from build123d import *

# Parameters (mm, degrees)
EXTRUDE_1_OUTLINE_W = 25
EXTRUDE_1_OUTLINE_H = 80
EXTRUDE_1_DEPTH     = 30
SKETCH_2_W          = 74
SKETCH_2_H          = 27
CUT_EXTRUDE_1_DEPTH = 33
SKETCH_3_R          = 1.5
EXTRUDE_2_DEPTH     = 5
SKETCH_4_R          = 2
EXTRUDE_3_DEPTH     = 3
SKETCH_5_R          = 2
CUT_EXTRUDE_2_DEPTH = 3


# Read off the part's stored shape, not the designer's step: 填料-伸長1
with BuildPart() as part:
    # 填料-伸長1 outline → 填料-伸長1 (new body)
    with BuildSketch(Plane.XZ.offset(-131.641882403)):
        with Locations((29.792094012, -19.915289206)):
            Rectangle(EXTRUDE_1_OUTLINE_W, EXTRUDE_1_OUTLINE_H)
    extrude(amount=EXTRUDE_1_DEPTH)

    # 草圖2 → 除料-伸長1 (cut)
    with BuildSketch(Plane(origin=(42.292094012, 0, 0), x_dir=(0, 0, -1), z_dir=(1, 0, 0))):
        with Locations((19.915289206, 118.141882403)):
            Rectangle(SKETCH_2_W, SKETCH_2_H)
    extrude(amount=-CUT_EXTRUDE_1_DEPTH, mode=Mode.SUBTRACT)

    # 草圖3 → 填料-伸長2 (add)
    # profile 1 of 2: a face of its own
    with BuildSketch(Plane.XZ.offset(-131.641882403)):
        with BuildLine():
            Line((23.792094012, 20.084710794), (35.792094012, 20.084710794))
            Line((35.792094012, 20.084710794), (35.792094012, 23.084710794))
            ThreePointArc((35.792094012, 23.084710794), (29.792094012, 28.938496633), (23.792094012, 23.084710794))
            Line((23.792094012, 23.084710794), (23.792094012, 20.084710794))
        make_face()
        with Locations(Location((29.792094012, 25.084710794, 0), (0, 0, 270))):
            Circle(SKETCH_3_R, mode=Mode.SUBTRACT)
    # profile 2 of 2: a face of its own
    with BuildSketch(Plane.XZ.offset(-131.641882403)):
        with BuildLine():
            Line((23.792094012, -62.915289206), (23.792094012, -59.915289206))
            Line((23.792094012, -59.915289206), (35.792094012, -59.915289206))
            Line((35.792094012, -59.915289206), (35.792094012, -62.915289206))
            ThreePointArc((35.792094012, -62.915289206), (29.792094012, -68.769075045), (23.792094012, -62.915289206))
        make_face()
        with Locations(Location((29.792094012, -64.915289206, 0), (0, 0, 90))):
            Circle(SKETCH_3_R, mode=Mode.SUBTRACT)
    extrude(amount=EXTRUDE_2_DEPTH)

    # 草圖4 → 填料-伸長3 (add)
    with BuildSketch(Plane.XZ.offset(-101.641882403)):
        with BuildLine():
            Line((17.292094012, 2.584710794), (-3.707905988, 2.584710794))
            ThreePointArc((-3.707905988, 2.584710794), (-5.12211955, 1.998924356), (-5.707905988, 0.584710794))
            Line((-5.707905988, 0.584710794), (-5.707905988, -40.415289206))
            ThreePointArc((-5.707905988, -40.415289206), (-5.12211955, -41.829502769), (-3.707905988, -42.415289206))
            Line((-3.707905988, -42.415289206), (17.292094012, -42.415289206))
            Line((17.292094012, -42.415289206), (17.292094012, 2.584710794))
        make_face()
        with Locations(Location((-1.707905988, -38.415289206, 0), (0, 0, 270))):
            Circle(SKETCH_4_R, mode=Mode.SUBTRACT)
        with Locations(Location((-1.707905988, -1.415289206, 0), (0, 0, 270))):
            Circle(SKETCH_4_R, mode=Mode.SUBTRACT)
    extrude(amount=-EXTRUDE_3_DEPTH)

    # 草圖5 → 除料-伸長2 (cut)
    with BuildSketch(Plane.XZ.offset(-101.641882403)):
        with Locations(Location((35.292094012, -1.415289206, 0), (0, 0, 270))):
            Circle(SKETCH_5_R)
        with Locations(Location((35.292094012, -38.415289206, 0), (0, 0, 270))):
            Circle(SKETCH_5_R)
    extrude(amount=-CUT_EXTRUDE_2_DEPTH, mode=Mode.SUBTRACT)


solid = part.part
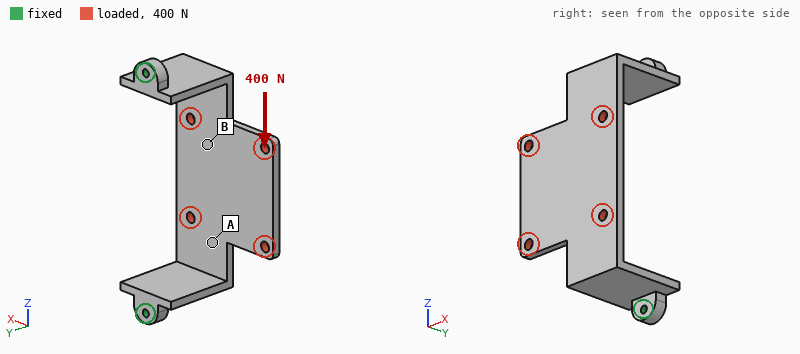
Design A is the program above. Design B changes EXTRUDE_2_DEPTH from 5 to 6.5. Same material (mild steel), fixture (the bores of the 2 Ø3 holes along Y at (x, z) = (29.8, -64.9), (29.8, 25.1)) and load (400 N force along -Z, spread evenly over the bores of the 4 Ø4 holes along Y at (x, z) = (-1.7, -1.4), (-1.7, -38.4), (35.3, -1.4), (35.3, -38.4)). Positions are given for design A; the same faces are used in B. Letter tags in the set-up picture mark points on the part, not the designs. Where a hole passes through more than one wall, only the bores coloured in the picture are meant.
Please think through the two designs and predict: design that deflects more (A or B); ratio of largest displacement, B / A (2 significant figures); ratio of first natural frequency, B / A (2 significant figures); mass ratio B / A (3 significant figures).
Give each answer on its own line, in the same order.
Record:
A
0.75
1.1
1.02
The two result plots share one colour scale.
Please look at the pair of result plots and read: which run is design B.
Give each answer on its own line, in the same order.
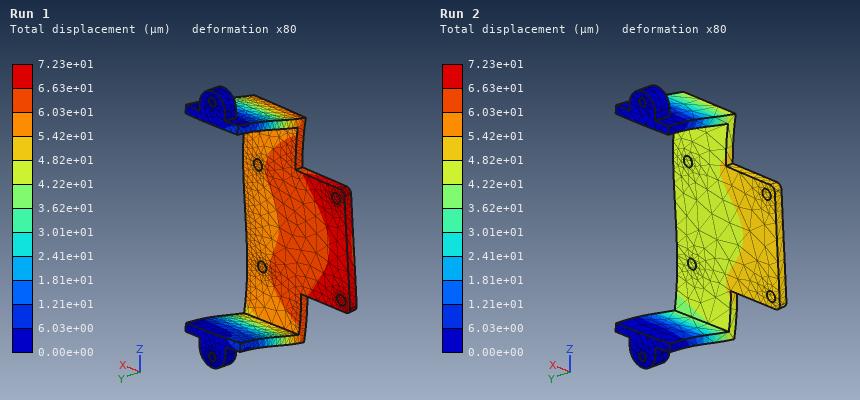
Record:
Run 2
